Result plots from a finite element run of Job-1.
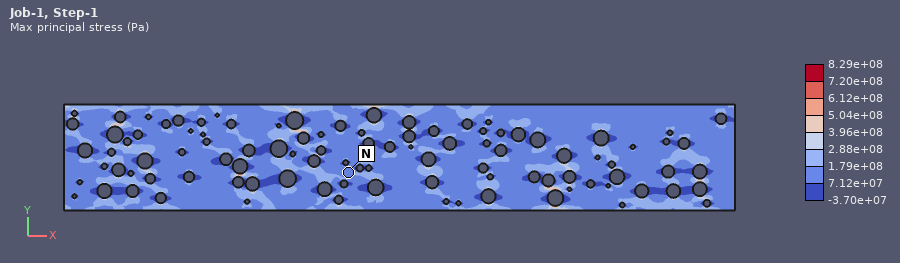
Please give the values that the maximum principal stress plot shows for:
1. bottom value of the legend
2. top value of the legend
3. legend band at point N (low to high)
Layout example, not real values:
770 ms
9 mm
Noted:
-3.70e+07 Pa
8.29e+08 Pa
7.12e+07 to 1.79e+08 Pa
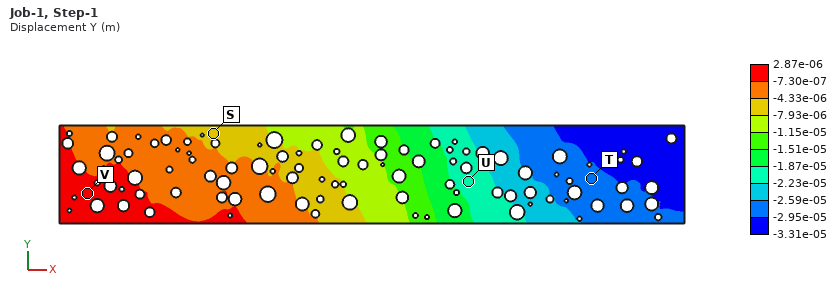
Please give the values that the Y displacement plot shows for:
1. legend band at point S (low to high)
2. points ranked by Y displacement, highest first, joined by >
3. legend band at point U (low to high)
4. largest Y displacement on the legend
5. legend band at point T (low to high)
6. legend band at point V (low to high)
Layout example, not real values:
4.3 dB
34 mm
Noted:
-7.93e-06 to -4.33e-06 m
V > S > U > T
-2.23e-05 to -1.87e-05 m
2.87e-06 m
-2.95e-05 to -2.59e-05 m
-7.30e-07 to 2.87e-06 m
